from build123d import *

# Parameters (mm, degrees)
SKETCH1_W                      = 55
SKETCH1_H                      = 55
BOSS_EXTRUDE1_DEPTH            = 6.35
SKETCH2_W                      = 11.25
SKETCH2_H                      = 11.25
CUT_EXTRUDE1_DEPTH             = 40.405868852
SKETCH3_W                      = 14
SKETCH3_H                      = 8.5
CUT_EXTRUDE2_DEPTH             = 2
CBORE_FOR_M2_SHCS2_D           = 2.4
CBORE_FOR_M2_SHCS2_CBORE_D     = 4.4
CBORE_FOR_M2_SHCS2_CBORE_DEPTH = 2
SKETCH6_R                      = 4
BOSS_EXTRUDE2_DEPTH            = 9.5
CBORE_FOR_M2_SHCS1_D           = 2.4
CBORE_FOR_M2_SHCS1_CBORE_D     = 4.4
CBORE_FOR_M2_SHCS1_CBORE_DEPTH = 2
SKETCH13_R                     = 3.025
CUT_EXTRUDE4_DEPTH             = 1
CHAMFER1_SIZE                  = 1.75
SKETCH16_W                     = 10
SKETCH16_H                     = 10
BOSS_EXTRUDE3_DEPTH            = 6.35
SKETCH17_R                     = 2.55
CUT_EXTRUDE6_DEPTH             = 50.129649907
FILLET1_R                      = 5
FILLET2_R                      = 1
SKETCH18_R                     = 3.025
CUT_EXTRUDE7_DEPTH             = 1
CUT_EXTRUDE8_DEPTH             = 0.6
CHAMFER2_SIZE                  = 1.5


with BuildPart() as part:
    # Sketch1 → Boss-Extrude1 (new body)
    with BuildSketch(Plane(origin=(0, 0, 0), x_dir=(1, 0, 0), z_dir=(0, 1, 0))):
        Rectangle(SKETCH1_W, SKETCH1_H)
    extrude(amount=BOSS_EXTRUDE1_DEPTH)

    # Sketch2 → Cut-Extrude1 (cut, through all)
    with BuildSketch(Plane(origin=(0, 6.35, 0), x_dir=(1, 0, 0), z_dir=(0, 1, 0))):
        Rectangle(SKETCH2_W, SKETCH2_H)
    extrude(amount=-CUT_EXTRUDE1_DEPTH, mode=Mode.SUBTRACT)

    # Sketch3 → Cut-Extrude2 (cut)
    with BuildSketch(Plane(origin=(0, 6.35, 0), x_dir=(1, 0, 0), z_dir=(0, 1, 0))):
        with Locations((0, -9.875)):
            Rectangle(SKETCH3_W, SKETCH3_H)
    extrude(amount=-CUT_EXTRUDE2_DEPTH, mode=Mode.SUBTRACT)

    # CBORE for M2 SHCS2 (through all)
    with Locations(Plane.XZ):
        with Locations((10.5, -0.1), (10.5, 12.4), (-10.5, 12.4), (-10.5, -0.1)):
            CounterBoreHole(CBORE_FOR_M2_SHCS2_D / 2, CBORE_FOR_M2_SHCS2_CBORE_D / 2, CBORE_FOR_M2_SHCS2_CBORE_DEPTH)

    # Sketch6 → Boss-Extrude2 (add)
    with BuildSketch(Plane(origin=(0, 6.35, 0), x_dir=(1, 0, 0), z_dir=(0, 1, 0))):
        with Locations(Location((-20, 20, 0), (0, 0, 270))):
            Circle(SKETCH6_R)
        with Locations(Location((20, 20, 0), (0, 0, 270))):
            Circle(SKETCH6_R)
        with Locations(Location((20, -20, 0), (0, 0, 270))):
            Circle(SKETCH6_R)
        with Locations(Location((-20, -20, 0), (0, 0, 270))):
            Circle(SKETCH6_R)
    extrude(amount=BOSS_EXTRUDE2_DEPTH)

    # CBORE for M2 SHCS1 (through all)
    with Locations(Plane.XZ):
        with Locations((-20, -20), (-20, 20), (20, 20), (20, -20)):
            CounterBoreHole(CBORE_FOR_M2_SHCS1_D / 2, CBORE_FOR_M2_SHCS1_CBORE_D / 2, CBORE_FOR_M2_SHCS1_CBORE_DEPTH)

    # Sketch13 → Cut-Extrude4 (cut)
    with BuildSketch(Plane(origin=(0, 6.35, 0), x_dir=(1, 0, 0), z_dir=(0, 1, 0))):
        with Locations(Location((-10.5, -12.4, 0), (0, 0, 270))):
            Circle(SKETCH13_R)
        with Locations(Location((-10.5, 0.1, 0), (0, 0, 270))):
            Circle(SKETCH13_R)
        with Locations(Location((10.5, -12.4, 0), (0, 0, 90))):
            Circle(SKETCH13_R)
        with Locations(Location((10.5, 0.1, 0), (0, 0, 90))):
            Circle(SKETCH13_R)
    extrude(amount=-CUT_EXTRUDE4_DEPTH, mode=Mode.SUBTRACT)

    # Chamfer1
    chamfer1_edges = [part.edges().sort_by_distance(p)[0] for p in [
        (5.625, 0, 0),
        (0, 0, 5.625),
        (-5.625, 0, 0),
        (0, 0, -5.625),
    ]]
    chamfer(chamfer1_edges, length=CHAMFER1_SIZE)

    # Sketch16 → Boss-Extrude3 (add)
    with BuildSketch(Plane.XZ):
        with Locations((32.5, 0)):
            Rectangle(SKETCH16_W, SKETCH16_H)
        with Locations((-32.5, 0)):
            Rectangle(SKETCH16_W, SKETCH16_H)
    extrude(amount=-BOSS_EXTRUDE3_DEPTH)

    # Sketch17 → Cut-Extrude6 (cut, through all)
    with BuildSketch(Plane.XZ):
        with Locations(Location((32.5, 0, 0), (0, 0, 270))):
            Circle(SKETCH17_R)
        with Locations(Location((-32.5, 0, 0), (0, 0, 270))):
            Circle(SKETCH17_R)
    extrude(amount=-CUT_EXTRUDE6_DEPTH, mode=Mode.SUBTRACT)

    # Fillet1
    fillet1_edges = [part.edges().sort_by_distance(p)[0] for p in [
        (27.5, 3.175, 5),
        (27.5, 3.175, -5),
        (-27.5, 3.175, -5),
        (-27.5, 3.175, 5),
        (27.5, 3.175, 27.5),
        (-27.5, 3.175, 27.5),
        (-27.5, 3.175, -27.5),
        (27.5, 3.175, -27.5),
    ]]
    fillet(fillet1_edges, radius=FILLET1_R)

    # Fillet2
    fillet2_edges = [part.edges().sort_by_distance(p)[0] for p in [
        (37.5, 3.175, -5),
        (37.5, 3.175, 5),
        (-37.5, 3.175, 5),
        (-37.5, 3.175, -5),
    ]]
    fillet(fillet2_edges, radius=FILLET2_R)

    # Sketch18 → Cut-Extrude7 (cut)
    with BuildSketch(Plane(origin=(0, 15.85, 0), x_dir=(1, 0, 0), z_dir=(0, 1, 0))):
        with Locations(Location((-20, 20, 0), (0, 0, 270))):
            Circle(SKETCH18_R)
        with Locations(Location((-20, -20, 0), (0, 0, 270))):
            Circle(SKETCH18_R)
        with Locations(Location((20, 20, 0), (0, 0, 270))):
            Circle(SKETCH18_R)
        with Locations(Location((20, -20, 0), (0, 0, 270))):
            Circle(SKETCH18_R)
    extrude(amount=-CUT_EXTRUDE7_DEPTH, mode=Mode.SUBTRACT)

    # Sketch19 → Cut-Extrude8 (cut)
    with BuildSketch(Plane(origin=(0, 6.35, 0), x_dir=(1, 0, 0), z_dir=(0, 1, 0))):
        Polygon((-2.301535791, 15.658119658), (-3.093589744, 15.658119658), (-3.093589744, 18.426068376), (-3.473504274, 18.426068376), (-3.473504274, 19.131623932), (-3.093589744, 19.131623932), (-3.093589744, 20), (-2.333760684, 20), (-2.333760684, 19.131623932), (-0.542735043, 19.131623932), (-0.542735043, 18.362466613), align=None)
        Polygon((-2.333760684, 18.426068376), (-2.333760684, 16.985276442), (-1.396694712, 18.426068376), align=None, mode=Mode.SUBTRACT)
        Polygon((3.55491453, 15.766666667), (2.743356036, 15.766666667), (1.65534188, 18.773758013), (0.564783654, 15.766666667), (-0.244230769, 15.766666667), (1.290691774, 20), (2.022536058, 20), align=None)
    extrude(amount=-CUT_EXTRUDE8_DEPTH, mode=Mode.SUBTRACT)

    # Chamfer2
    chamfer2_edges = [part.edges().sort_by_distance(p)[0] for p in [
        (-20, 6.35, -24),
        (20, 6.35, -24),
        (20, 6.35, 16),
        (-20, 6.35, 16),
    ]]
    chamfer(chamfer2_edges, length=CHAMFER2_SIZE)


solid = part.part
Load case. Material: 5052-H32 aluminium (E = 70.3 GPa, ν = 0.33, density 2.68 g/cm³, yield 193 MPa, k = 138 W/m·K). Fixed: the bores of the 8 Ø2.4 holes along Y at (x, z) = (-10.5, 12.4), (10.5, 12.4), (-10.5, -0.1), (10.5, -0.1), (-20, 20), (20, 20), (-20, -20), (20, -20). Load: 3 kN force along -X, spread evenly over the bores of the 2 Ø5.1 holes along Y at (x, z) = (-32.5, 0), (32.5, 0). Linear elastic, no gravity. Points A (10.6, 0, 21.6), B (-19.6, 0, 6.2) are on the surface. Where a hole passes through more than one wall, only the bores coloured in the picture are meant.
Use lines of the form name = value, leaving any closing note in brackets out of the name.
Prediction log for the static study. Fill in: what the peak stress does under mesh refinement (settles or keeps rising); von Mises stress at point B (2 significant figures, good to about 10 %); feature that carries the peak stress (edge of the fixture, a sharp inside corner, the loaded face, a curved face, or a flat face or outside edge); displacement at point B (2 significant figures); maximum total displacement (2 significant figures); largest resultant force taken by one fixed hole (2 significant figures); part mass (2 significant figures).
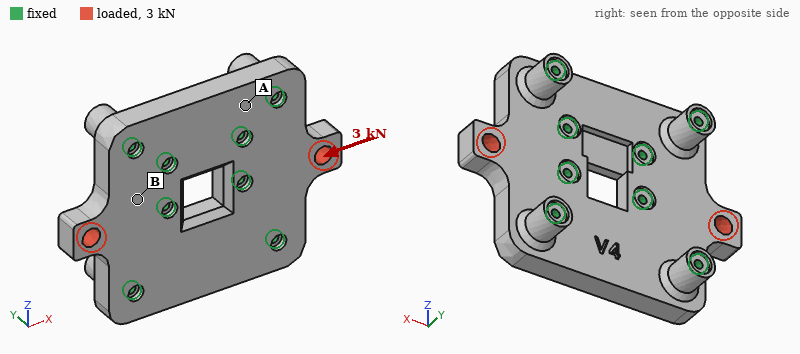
what the peak stress does under mesh refinement = keeps rising
von Mises stress at point B = 10 MPa
feature that carries the peak stress = edge of the fixture
displacement at point B = 1.9 µm
maximum total displacement = 7.6 µm
largest resultant force taken by one fixed hole = 650 N
part mass = 55 g
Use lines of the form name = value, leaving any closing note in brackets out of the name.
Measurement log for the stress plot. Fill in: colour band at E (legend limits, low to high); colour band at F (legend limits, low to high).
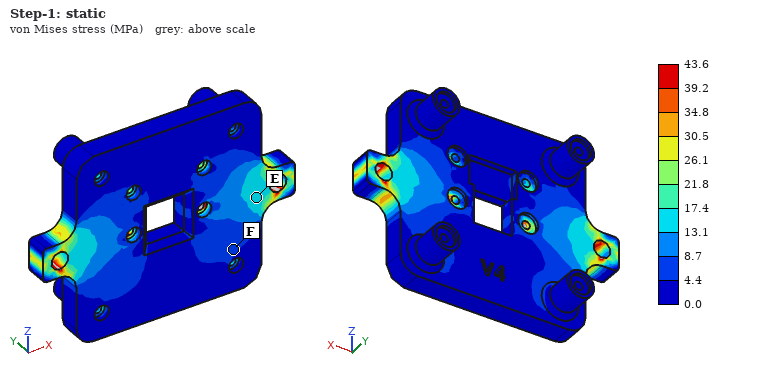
colour band at E = 13.1 to 17.4 MPa
colour band at F = 4.4 to 8.7 MPa
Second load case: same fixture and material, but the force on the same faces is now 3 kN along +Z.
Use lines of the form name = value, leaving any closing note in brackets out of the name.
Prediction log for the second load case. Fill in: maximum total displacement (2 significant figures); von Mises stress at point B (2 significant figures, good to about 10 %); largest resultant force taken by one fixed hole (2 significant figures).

maximum total displacement = 22 µm
von Mises stress at point B = 8.7 MPa
largest resultant force taken by one fixed hole = 680 N
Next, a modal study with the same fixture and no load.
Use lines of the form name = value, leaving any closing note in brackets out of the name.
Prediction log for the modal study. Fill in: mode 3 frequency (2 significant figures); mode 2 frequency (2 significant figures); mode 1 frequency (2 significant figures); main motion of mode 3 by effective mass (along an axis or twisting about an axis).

mode 3 frequency = 20 kHz
mode 2 frequency = 14 kHz
mode 1 frequency = 14 kHz
main motion of mode 3 by effective mass = along Y
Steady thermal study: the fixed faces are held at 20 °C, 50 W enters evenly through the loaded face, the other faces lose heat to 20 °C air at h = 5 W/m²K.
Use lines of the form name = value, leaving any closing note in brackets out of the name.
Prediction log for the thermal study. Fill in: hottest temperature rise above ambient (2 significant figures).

hottest temperature rise above ambient = 40 K
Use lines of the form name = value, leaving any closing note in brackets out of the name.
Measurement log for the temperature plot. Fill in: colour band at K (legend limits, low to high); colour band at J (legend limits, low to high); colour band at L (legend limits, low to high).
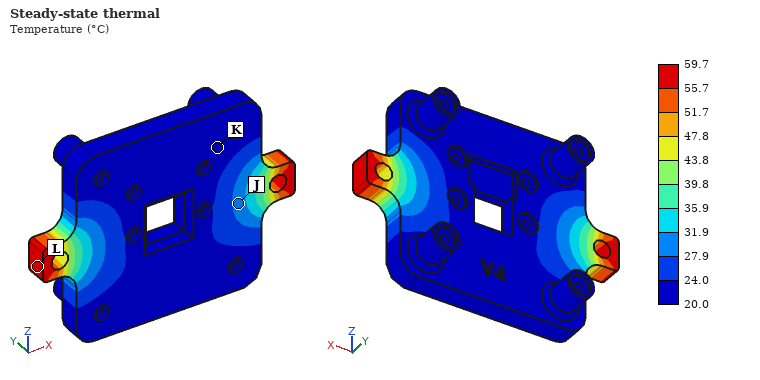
colour band at K = 20.0 to 24.0 °C
colour band at J = 27.9 to 31.9 °C
colour band at L = 55.7 to 59.7 °C
